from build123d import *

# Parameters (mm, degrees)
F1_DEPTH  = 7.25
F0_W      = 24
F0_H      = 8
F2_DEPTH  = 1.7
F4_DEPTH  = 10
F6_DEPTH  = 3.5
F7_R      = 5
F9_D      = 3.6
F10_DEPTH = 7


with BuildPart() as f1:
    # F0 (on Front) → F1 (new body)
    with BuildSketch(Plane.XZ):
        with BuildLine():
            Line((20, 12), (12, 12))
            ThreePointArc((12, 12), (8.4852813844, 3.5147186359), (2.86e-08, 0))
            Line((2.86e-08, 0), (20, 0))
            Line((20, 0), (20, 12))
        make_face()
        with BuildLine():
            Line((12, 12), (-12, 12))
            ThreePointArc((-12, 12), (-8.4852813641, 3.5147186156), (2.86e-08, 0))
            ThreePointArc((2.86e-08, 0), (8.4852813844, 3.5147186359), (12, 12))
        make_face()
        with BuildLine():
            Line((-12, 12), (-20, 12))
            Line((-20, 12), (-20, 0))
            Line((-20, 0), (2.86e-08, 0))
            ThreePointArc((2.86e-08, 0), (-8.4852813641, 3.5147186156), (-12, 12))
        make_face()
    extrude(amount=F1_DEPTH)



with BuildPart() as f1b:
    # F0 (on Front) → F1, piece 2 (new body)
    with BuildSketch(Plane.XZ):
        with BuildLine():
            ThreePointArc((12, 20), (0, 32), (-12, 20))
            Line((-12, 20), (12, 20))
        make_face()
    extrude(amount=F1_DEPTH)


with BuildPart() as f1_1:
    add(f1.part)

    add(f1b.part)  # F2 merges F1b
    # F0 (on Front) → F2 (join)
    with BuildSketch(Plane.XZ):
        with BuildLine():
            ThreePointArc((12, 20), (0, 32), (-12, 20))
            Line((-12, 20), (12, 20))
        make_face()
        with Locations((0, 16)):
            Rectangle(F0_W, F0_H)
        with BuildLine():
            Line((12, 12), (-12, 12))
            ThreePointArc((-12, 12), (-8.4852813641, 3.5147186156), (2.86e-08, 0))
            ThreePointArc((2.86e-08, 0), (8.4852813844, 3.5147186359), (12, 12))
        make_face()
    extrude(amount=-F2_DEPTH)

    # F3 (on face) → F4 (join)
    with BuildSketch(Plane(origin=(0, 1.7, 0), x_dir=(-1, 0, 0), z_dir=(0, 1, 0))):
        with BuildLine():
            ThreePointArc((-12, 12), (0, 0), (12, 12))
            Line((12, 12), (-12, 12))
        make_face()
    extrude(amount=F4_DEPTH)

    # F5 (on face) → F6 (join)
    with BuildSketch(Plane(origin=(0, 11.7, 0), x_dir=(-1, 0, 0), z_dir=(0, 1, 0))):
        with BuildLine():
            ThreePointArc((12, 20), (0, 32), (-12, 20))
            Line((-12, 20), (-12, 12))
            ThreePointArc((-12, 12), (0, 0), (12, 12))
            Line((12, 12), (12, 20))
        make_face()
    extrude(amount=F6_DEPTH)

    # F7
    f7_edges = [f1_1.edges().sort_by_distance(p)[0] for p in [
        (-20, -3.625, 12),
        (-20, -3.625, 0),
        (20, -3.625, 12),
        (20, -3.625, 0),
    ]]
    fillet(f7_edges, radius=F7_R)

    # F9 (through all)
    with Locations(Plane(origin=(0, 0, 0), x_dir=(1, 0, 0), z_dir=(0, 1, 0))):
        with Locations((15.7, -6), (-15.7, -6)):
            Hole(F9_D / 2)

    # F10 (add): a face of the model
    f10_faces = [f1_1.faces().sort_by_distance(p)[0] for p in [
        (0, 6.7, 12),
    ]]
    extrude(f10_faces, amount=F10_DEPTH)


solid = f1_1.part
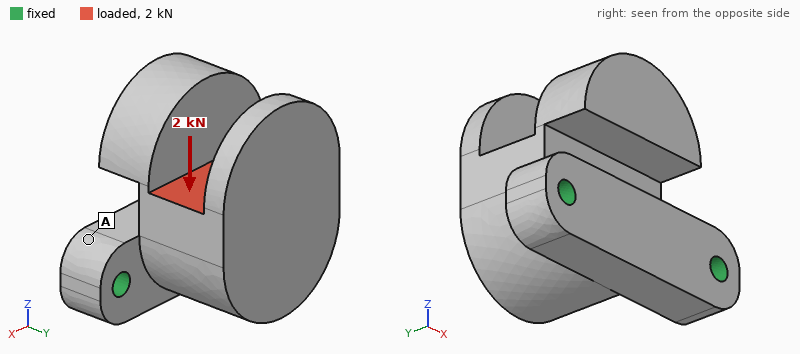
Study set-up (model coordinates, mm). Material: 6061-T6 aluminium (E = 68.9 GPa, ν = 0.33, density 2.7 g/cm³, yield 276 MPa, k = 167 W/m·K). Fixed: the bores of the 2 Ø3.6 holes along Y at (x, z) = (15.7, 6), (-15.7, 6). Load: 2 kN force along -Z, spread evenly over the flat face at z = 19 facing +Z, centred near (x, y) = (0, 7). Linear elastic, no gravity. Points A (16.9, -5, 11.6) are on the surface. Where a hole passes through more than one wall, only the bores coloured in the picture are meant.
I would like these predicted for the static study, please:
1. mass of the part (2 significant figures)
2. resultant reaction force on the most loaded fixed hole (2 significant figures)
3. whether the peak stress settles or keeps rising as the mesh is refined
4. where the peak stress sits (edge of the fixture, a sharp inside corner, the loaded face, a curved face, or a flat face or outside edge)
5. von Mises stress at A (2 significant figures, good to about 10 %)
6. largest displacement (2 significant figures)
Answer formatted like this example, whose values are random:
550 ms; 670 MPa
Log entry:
33 g; 1.0 kN; keeps rising; edge of the fixture; 28 MPa; 0.11 mm
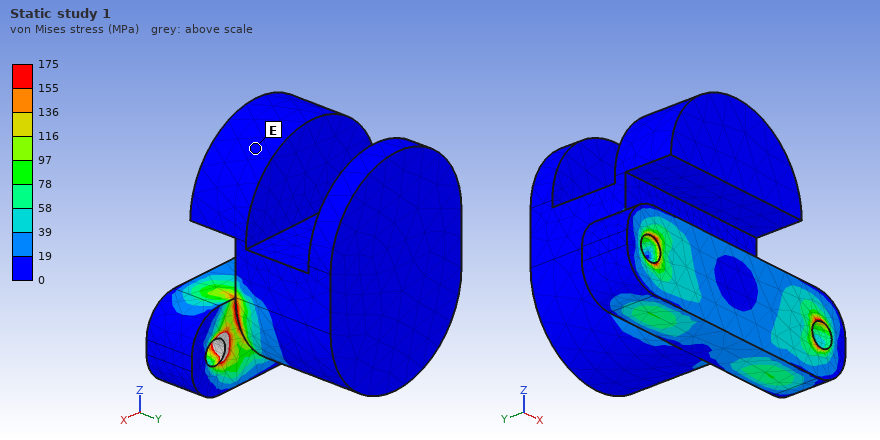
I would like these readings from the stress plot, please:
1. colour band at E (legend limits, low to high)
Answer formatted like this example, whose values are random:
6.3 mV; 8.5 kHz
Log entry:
0 to 19 MPa
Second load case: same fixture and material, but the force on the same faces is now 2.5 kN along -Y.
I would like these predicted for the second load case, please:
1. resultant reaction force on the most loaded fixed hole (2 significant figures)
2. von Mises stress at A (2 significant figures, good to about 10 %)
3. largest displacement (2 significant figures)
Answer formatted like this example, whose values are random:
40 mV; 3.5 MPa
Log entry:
1.3 kN; 45 MPa; 0.19 mm
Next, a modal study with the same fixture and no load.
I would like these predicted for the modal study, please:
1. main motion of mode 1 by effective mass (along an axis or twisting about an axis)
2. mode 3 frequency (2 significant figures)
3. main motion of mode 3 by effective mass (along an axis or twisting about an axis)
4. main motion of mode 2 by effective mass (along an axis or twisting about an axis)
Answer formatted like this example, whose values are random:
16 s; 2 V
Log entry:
along Y; 12 kHz; along X; along Z
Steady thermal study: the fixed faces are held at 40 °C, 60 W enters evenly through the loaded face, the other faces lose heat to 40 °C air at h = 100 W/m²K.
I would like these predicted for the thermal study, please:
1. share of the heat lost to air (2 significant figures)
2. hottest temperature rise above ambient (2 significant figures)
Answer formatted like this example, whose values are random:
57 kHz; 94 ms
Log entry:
15 %; 32 K
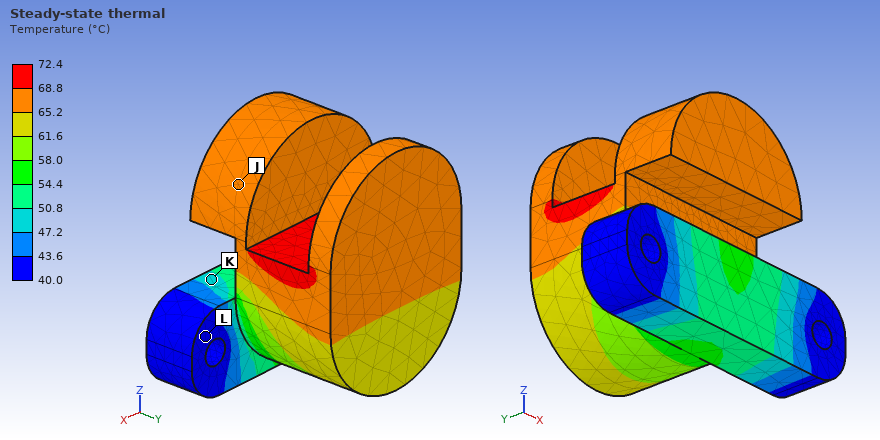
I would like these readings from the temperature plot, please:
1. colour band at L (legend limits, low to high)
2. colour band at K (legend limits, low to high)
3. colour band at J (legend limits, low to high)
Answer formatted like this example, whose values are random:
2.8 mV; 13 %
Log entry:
40.0 to 43.6 °C; 47.2 to 50.8 °C; 65.2 to 68.8 °C
